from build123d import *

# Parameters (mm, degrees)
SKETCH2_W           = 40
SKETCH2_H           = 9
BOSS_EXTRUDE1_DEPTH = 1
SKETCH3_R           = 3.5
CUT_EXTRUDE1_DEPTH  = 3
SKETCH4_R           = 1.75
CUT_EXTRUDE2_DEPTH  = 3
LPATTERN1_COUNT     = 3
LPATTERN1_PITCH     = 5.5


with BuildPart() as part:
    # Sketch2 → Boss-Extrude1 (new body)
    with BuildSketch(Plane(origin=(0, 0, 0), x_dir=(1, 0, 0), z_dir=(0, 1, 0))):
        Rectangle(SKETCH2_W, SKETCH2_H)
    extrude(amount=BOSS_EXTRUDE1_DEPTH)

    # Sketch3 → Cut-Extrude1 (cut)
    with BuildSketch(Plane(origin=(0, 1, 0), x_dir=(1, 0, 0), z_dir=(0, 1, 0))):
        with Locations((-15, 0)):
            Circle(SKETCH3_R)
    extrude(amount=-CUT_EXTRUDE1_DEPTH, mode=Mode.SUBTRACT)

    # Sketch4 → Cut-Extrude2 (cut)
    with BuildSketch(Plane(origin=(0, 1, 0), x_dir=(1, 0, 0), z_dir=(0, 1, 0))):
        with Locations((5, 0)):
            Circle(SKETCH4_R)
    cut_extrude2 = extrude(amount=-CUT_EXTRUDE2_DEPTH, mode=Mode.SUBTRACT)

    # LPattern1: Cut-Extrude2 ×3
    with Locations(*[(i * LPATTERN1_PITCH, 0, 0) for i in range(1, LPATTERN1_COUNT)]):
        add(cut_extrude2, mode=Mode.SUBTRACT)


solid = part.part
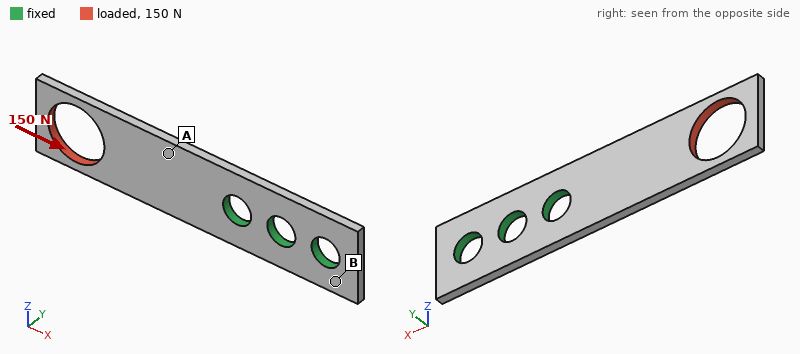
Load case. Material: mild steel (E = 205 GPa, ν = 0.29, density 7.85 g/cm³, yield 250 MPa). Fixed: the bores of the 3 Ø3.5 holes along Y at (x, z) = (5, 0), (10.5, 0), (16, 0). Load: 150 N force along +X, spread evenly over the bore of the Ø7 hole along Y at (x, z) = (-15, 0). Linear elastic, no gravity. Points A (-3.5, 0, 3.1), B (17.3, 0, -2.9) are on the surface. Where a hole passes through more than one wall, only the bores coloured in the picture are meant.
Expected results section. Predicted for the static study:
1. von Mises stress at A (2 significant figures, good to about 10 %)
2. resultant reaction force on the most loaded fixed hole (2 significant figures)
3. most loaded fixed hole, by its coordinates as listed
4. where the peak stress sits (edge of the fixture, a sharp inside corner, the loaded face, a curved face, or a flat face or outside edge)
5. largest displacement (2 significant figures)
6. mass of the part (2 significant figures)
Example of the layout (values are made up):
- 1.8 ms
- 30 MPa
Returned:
- 17 MPa
- 130 N
- (5, 0)
- the loaded face
- 5.1 µm
- 2.3 g
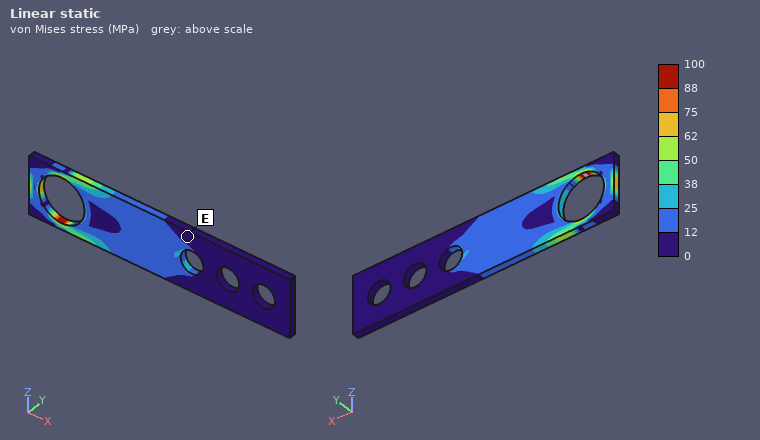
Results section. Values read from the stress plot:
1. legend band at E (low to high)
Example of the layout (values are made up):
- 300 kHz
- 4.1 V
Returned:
- 0 to 12 MPa
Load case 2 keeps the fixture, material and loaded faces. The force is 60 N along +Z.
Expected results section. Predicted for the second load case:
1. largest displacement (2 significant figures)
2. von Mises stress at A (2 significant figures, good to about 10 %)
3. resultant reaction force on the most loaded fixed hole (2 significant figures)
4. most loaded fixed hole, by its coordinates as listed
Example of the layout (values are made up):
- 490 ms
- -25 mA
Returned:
- 31 µm
- 37 MPa
- 120 N
- (5, 0)
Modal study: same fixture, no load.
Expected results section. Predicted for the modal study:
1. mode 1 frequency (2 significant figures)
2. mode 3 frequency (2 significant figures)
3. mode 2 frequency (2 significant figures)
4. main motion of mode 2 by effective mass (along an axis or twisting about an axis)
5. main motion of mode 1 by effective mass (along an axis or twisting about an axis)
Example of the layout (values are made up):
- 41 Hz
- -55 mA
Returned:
- 1800 Hz
- 8000 Hz
- 7500 Hz
- twisting about X
- along Y
